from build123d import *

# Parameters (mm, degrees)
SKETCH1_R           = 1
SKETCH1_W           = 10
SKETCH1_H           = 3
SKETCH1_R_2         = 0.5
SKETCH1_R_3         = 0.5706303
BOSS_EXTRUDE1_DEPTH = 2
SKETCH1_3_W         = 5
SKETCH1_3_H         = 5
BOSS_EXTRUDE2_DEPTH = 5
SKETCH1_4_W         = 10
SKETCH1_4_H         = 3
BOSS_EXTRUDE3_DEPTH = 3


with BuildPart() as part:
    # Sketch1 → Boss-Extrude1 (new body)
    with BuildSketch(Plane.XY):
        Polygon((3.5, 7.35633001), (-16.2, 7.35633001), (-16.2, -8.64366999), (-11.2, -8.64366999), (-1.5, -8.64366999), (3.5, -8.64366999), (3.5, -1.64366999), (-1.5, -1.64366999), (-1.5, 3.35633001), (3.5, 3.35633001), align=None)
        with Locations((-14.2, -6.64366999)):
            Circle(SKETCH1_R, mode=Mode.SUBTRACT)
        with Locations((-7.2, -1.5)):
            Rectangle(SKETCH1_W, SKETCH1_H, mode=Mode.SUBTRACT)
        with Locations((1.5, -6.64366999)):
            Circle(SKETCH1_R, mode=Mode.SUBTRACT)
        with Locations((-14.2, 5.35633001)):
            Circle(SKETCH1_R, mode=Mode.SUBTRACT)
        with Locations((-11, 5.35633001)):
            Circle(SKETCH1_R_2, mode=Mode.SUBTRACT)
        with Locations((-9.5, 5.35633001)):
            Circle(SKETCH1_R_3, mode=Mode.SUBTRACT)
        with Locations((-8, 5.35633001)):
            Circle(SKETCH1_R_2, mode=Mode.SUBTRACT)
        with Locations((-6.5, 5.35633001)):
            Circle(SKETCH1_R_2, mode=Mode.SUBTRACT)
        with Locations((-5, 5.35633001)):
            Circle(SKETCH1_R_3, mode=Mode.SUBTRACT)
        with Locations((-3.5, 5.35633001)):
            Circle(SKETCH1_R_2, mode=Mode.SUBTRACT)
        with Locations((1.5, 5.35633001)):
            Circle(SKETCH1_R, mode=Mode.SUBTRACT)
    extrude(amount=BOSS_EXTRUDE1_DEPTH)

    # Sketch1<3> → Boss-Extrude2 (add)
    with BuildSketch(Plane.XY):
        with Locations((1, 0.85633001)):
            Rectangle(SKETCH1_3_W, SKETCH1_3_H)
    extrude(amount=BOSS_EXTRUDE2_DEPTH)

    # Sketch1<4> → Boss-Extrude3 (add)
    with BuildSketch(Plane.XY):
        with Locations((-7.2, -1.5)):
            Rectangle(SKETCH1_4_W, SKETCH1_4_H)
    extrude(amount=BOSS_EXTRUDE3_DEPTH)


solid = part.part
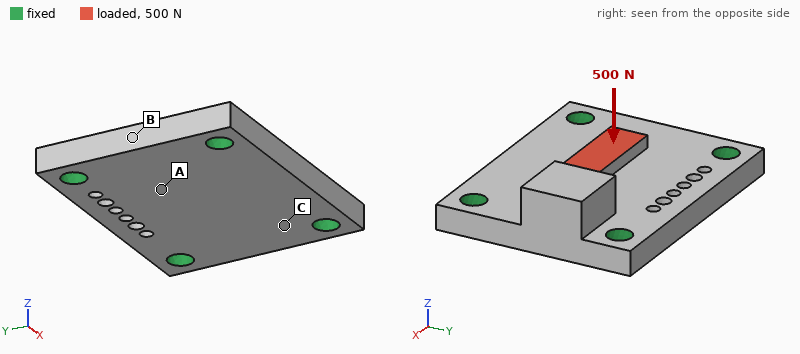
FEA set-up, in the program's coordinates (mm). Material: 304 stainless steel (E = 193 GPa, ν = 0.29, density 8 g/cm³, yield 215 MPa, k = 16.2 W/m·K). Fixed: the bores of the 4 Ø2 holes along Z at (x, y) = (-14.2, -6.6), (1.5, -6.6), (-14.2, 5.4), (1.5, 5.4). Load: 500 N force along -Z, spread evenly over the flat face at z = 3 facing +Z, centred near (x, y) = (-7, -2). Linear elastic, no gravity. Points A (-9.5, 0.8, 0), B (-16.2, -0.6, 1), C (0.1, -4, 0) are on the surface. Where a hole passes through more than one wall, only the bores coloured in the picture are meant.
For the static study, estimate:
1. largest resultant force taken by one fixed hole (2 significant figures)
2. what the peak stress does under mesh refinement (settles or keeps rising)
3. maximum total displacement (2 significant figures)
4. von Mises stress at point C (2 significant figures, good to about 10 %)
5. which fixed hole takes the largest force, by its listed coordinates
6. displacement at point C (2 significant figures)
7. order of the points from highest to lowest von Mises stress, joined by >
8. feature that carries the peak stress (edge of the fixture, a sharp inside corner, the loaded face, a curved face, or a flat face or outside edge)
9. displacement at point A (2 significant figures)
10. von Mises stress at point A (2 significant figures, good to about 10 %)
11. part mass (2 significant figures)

160 N
keeps rising
5.7 µm
30 MPa
(-14.2, -6.6)
1.6 µm
A > C > B
edge of the fixture
4.6 µm
46 MPa
5.6 g
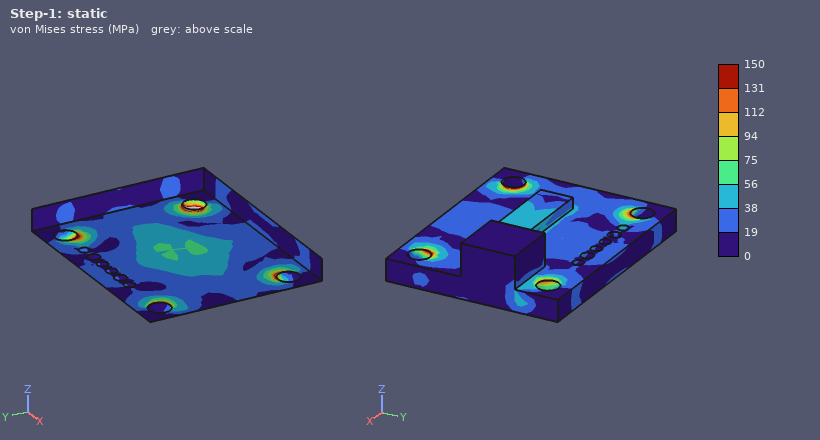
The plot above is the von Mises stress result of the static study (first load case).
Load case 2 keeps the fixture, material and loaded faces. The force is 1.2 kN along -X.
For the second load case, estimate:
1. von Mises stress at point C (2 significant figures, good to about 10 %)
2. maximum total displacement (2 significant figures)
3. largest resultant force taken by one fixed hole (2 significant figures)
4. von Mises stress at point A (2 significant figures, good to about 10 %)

43 MPa
4.1 µm
400 N
14 MPa
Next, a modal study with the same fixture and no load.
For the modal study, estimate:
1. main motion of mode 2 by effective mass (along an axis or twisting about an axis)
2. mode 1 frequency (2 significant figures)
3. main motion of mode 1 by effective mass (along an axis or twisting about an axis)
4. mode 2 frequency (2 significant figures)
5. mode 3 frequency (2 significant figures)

twisting about X
34 kHz
along Z
49 kHz
56 kHz
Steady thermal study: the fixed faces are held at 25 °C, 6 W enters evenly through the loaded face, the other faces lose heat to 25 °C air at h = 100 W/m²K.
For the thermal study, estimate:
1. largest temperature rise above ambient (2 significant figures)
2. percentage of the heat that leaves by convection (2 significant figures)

61 K
22 %
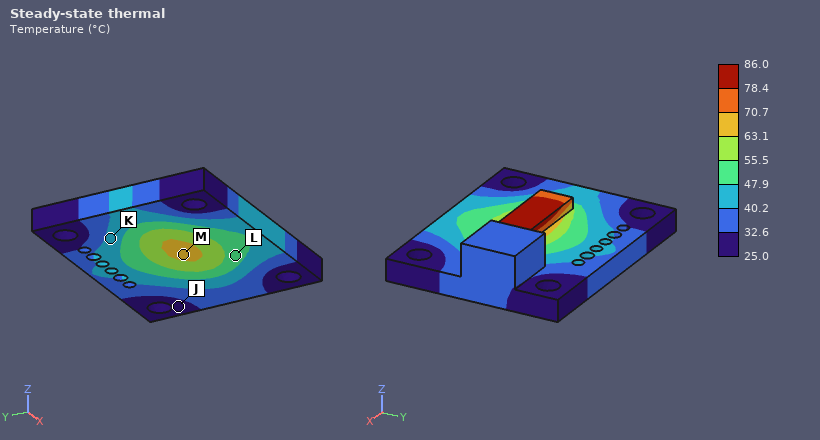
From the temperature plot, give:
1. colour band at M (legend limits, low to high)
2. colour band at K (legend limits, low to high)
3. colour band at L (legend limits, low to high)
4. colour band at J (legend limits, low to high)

63.1 to 70.7 °C
40.2 to 47.9 °C
47.9 to 55.5 °C
25.0 to 32.6 °C
